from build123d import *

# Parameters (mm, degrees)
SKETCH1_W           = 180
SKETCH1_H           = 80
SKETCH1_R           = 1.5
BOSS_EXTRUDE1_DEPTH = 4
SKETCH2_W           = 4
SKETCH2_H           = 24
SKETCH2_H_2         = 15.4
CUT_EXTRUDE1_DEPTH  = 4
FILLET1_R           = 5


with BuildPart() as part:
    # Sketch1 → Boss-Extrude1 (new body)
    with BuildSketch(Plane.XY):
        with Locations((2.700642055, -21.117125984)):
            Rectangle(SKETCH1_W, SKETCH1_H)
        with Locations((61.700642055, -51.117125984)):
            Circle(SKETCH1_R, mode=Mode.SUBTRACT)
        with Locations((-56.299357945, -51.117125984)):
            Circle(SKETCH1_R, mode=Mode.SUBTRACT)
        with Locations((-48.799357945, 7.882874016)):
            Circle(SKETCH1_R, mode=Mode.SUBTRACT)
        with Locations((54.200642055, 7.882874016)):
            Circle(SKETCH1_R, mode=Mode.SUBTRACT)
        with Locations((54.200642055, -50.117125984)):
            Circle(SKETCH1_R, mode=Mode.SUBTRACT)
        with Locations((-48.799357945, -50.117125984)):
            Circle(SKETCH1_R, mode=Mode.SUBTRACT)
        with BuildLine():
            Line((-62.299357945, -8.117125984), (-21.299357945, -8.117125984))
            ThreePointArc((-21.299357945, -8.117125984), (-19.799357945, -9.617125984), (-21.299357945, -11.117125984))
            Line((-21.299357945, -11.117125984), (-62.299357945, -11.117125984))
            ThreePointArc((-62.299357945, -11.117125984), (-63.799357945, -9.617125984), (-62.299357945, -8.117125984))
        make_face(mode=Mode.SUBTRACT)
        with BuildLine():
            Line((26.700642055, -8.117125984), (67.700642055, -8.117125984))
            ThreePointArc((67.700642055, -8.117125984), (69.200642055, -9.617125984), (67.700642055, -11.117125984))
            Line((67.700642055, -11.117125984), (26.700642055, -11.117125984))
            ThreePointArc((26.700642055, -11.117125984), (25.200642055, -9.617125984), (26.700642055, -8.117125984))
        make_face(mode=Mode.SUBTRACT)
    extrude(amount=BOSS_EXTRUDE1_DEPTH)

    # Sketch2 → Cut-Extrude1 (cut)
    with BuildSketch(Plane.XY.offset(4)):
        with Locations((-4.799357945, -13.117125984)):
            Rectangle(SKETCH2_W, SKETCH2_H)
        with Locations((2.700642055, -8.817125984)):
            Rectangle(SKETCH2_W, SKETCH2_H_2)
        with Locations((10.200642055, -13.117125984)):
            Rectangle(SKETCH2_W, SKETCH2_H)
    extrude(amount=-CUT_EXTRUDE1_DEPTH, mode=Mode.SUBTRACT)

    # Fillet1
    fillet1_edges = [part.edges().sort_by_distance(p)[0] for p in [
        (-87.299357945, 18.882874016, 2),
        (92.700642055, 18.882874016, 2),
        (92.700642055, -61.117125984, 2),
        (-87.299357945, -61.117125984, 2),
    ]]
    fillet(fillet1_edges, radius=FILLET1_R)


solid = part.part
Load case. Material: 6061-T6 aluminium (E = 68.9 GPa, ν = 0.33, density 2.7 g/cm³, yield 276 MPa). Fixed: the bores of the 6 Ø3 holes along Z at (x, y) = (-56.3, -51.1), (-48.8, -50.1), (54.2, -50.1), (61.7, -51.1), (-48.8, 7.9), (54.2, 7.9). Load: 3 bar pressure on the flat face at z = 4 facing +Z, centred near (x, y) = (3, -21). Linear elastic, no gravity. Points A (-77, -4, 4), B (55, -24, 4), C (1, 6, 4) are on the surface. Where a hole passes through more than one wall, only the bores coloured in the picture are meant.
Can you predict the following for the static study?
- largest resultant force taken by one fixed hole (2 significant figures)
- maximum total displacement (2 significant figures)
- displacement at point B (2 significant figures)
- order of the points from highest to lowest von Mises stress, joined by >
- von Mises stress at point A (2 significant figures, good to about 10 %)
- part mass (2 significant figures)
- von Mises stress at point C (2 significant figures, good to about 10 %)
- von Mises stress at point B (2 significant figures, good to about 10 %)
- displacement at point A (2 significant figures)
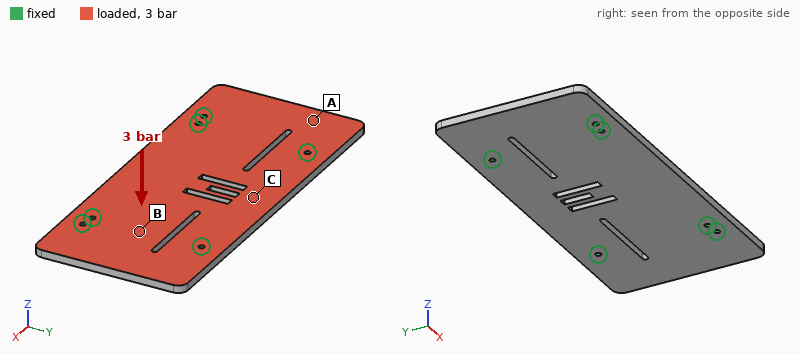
970 N
0.35 mm
0.086 mm
C > B > A
19 MPa
150 g
65 MPa
44 MPa
0.14 mm
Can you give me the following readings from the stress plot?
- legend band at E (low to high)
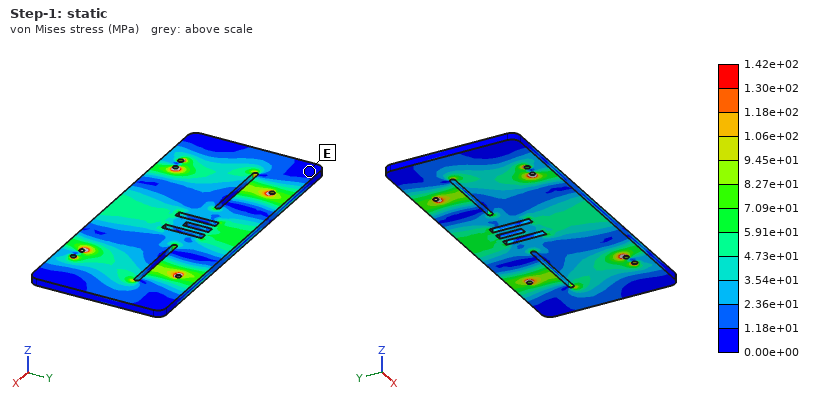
0.00e+00 to 1.18e+01 MPa
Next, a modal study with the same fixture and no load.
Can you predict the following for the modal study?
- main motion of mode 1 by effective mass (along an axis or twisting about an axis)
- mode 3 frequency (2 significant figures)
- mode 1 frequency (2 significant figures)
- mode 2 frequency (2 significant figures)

along Z
2100 Hz
1600 Hz
2100 Hz
